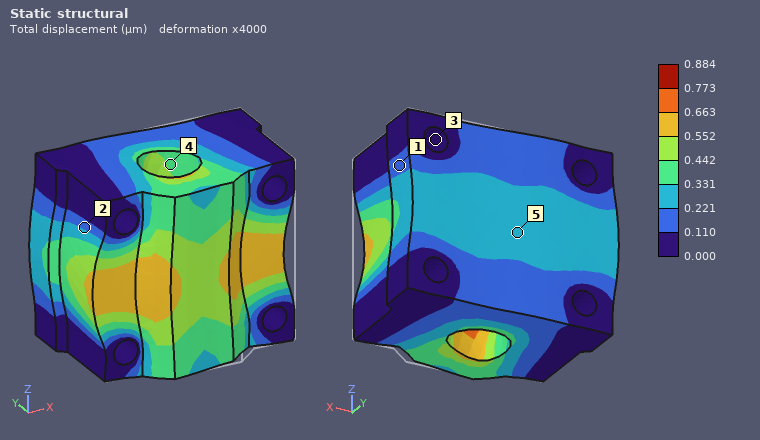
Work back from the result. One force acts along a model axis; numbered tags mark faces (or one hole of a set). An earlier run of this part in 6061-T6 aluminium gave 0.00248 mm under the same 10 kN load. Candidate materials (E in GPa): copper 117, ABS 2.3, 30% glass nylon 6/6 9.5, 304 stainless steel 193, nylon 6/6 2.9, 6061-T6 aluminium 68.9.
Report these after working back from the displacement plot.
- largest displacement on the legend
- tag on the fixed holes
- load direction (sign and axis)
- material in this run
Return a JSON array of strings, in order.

["0.884 µm", "3", "-X", "304 stainless steel"]
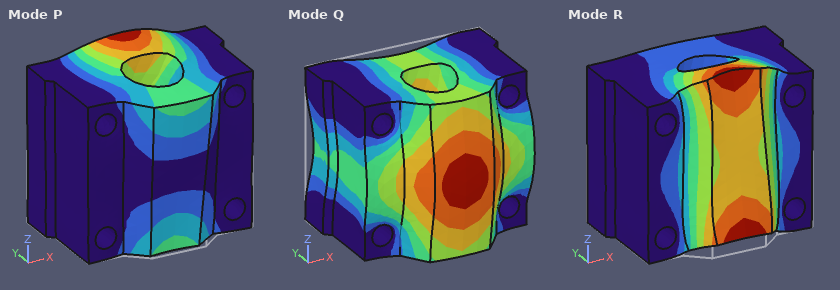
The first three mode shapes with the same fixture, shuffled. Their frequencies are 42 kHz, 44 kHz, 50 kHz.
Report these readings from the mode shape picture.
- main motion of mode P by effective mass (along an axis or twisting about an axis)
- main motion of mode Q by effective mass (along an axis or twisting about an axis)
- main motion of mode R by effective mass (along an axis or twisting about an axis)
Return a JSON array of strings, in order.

["along Z", "along Y", "along Z"]
